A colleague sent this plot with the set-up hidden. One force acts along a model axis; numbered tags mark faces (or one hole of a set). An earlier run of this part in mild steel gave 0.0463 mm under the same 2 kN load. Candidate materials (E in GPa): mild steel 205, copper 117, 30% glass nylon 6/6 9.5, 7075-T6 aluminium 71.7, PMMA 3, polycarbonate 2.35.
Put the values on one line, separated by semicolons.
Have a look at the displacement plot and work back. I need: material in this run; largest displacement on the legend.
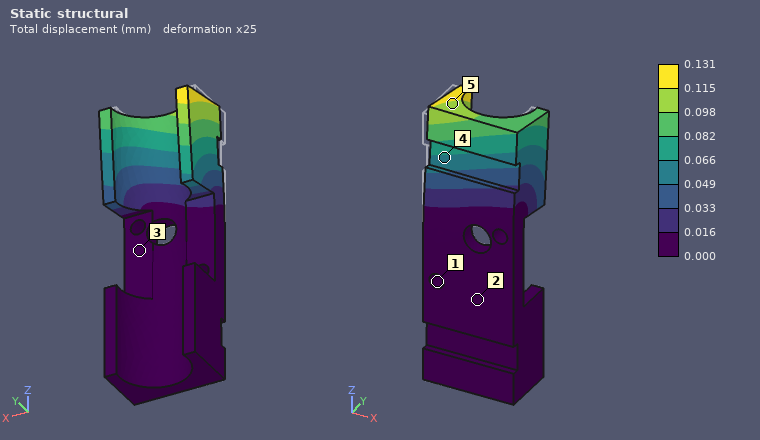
7075-T6 aluminium; 0.131 mm
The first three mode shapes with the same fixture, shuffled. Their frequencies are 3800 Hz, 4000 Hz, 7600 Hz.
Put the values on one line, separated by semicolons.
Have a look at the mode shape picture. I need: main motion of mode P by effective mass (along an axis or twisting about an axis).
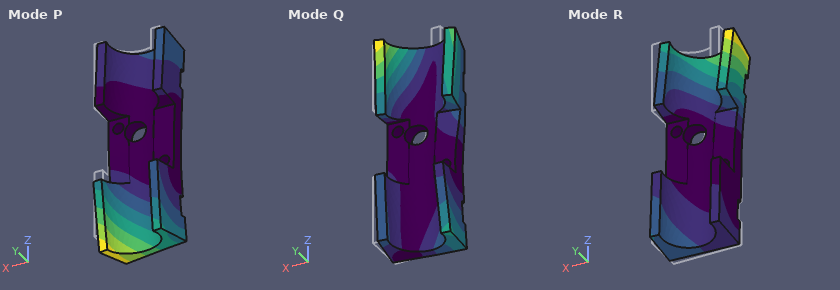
along Y
